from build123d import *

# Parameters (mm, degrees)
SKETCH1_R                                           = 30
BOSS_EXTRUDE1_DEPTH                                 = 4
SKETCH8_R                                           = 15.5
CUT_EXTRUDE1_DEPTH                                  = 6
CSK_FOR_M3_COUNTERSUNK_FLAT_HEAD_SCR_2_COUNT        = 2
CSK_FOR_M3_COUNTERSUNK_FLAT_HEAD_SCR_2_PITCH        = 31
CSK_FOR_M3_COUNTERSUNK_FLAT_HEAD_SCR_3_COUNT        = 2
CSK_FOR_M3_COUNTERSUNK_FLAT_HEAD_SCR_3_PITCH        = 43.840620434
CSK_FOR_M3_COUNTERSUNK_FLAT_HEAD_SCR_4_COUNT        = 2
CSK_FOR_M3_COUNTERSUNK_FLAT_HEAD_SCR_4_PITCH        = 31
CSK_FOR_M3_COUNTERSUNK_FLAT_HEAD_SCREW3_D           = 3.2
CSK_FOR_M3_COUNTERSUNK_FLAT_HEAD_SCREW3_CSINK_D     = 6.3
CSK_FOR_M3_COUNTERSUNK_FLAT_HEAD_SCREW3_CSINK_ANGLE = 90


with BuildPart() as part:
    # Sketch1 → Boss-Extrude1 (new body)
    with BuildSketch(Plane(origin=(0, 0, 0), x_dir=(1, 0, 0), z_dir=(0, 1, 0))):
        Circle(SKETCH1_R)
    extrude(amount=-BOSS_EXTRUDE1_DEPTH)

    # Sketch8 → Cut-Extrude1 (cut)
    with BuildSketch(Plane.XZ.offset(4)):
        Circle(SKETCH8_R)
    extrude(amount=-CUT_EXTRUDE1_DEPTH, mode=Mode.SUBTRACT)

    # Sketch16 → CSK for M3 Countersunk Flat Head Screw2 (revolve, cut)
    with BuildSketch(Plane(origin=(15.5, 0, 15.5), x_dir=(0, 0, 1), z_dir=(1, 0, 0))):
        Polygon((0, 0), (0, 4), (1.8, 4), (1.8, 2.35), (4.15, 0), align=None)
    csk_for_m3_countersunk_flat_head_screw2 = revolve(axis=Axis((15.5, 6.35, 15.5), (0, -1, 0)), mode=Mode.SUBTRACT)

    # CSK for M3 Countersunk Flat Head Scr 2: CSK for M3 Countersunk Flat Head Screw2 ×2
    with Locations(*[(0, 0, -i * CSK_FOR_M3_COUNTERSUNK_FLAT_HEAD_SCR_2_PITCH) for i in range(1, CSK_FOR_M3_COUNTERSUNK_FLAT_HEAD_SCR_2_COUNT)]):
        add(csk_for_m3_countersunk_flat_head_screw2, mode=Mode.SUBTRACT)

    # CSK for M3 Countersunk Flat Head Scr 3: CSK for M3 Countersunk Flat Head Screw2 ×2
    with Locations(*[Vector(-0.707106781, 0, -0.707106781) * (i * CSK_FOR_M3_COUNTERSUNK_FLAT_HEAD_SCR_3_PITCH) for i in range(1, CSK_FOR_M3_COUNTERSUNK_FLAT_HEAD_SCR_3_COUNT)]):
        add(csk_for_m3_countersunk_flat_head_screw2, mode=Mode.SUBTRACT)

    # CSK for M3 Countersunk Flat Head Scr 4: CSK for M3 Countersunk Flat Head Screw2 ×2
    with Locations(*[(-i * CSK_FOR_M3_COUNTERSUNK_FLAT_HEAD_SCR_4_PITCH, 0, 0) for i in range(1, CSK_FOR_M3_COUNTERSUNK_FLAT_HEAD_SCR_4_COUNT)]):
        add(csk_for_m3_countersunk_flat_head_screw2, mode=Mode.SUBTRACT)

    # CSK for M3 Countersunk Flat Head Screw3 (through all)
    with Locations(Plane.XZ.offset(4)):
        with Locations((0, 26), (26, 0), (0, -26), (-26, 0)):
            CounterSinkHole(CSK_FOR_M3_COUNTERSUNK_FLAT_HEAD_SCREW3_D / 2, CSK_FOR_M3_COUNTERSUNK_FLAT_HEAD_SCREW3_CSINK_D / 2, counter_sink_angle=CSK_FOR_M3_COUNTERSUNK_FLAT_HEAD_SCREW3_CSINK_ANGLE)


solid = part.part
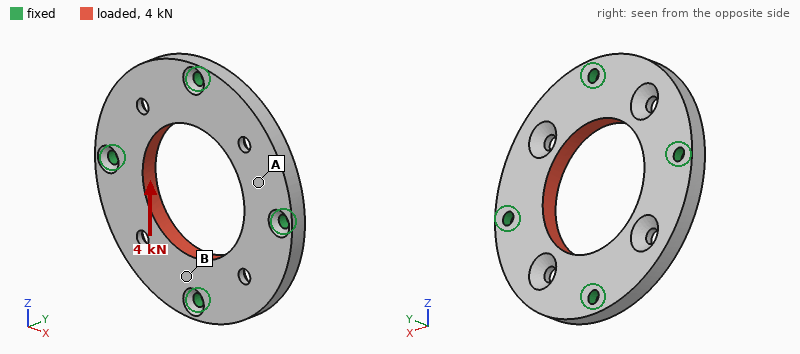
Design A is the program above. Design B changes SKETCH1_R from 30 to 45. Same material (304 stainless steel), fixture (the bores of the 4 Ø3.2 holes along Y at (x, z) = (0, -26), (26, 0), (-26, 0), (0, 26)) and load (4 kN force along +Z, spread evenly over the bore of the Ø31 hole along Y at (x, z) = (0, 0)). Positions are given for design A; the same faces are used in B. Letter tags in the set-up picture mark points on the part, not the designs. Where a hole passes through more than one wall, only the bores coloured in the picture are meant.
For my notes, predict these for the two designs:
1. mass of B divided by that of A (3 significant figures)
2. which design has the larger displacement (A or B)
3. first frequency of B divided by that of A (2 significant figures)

2.82
A
0.39
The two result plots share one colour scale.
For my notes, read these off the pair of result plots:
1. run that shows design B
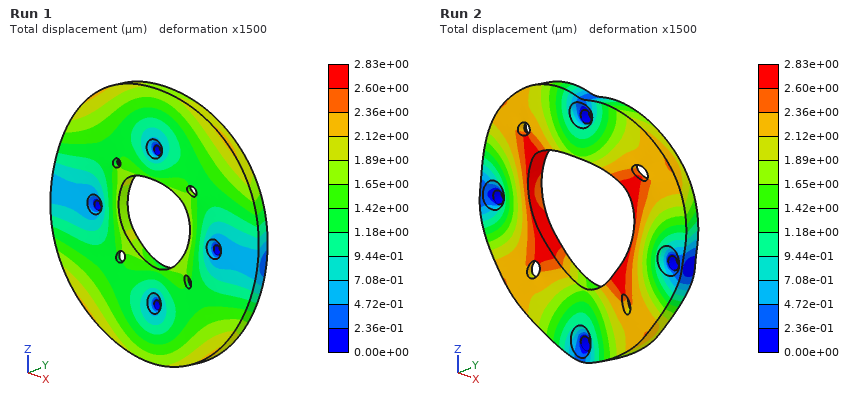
Run 1
